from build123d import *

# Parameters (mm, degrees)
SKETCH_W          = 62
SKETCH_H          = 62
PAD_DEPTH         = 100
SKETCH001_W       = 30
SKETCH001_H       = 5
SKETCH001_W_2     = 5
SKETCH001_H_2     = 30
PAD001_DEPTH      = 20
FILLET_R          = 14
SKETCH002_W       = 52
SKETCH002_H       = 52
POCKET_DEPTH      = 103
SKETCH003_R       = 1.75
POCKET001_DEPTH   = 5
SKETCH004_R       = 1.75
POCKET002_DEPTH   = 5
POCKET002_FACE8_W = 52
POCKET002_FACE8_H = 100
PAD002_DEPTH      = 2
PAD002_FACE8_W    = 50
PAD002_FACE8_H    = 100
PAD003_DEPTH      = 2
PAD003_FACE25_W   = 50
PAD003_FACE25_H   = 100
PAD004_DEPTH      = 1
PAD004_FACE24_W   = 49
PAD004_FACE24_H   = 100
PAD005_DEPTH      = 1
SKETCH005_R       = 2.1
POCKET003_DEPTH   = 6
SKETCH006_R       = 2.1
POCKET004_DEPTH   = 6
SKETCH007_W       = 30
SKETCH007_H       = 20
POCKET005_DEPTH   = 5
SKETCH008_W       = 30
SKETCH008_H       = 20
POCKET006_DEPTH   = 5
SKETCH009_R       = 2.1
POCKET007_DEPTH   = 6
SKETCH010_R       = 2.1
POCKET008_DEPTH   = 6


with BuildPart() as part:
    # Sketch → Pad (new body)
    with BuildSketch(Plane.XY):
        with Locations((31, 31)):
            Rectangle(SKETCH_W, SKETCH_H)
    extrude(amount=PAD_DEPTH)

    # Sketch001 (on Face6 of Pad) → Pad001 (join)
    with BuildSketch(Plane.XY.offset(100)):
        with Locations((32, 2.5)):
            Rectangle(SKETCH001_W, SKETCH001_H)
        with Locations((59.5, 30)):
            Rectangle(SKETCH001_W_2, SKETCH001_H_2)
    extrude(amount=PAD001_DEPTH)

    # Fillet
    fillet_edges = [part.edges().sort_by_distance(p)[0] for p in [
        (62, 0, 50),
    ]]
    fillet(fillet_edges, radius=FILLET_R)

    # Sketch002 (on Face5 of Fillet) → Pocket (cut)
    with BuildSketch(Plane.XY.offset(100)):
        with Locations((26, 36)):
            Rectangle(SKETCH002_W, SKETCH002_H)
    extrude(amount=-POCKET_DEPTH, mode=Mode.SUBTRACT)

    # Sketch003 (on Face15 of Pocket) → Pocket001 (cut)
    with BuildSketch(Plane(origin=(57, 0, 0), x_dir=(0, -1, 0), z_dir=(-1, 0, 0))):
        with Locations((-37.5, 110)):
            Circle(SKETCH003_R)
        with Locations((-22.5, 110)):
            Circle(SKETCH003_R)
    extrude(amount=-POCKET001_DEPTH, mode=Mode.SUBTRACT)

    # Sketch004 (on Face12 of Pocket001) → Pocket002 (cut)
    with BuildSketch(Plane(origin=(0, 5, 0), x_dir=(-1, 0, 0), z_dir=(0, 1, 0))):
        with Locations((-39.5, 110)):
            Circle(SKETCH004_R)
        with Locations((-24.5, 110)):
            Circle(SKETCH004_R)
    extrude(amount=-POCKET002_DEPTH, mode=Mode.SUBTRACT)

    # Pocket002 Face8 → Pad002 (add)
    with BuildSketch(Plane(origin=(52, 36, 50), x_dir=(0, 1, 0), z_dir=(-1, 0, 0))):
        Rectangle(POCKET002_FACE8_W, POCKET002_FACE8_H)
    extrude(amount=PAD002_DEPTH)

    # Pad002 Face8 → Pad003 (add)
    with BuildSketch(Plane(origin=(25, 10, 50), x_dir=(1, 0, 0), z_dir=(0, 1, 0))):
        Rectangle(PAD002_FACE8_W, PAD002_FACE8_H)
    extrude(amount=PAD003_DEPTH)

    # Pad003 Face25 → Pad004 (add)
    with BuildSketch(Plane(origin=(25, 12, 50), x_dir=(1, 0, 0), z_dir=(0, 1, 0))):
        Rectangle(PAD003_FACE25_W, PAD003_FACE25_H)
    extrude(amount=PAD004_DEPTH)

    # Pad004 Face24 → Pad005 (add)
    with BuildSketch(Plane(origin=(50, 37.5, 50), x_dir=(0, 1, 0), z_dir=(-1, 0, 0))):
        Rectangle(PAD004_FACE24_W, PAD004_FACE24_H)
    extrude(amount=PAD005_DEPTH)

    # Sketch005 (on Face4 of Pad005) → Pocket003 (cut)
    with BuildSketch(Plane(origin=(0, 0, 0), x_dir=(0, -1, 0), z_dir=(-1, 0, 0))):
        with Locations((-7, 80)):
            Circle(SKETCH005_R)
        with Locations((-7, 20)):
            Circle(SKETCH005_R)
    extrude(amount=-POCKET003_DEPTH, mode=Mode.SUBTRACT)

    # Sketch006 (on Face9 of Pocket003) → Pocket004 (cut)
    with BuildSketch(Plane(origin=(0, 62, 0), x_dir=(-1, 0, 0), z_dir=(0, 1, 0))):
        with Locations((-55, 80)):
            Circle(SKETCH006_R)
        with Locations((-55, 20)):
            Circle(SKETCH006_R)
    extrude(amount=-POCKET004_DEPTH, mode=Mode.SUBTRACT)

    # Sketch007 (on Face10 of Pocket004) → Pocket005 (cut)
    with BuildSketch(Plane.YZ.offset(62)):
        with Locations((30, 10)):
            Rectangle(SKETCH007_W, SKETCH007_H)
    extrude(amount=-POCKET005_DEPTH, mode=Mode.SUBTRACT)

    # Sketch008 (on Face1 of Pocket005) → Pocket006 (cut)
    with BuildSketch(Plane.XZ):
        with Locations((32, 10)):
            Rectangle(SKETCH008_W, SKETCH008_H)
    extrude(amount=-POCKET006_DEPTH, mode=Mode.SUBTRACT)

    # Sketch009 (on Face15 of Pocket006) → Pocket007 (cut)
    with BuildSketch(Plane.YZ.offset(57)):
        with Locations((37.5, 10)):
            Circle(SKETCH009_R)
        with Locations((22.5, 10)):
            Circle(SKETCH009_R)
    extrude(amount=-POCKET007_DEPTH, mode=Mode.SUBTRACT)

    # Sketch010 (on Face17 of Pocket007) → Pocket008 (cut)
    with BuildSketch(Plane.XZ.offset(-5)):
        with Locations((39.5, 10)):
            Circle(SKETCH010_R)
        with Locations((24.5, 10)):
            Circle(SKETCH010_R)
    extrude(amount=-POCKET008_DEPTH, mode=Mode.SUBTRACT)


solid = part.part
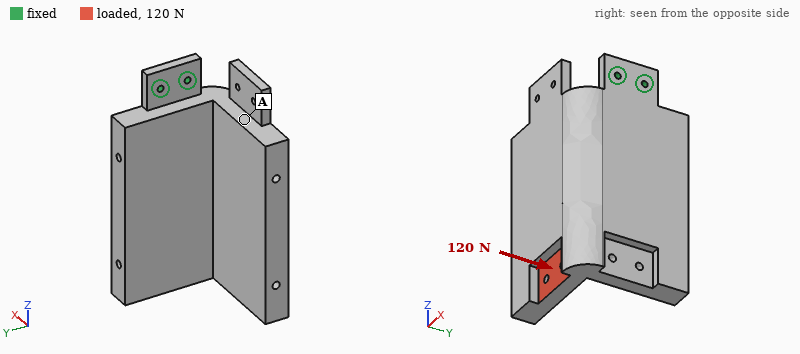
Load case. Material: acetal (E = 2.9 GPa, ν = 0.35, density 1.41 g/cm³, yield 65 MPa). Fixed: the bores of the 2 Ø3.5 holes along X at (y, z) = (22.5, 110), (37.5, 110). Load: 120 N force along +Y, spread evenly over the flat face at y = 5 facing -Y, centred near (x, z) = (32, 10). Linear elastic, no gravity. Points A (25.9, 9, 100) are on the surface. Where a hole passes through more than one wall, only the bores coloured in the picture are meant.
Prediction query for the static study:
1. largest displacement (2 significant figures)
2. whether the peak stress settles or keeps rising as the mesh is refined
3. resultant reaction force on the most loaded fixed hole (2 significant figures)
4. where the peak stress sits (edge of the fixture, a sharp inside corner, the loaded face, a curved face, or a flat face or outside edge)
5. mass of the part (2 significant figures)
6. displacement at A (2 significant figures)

1.6 mm
keeps rising
730 N
edge of the fixture
200 g
0.42 mm
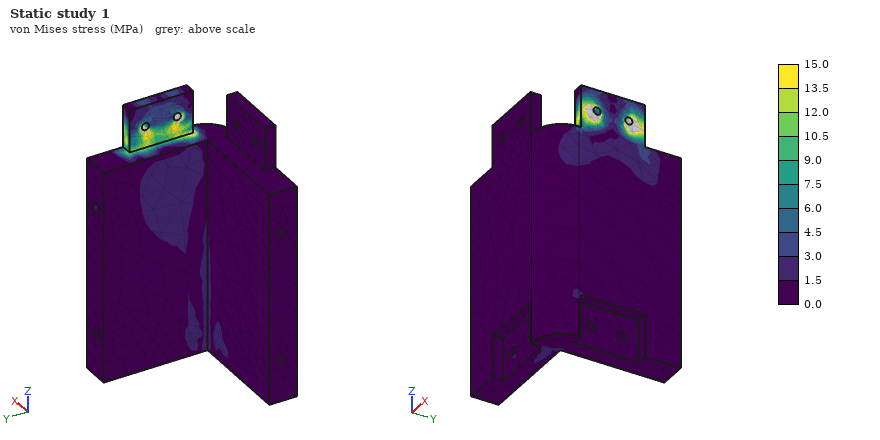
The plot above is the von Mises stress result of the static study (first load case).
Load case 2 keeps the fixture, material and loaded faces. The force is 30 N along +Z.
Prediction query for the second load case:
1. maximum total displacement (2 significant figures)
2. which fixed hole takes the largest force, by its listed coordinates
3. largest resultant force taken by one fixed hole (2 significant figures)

1.3 mm
(22.5, 110)
60 N
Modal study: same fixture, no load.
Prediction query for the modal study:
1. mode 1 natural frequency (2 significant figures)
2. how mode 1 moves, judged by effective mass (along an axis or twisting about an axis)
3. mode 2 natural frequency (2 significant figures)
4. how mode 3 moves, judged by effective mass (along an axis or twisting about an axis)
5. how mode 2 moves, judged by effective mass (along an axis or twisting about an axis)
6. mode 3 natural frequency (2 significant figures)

49 Hz
along X
170 Hz
along Y
along Y
260 Hz
